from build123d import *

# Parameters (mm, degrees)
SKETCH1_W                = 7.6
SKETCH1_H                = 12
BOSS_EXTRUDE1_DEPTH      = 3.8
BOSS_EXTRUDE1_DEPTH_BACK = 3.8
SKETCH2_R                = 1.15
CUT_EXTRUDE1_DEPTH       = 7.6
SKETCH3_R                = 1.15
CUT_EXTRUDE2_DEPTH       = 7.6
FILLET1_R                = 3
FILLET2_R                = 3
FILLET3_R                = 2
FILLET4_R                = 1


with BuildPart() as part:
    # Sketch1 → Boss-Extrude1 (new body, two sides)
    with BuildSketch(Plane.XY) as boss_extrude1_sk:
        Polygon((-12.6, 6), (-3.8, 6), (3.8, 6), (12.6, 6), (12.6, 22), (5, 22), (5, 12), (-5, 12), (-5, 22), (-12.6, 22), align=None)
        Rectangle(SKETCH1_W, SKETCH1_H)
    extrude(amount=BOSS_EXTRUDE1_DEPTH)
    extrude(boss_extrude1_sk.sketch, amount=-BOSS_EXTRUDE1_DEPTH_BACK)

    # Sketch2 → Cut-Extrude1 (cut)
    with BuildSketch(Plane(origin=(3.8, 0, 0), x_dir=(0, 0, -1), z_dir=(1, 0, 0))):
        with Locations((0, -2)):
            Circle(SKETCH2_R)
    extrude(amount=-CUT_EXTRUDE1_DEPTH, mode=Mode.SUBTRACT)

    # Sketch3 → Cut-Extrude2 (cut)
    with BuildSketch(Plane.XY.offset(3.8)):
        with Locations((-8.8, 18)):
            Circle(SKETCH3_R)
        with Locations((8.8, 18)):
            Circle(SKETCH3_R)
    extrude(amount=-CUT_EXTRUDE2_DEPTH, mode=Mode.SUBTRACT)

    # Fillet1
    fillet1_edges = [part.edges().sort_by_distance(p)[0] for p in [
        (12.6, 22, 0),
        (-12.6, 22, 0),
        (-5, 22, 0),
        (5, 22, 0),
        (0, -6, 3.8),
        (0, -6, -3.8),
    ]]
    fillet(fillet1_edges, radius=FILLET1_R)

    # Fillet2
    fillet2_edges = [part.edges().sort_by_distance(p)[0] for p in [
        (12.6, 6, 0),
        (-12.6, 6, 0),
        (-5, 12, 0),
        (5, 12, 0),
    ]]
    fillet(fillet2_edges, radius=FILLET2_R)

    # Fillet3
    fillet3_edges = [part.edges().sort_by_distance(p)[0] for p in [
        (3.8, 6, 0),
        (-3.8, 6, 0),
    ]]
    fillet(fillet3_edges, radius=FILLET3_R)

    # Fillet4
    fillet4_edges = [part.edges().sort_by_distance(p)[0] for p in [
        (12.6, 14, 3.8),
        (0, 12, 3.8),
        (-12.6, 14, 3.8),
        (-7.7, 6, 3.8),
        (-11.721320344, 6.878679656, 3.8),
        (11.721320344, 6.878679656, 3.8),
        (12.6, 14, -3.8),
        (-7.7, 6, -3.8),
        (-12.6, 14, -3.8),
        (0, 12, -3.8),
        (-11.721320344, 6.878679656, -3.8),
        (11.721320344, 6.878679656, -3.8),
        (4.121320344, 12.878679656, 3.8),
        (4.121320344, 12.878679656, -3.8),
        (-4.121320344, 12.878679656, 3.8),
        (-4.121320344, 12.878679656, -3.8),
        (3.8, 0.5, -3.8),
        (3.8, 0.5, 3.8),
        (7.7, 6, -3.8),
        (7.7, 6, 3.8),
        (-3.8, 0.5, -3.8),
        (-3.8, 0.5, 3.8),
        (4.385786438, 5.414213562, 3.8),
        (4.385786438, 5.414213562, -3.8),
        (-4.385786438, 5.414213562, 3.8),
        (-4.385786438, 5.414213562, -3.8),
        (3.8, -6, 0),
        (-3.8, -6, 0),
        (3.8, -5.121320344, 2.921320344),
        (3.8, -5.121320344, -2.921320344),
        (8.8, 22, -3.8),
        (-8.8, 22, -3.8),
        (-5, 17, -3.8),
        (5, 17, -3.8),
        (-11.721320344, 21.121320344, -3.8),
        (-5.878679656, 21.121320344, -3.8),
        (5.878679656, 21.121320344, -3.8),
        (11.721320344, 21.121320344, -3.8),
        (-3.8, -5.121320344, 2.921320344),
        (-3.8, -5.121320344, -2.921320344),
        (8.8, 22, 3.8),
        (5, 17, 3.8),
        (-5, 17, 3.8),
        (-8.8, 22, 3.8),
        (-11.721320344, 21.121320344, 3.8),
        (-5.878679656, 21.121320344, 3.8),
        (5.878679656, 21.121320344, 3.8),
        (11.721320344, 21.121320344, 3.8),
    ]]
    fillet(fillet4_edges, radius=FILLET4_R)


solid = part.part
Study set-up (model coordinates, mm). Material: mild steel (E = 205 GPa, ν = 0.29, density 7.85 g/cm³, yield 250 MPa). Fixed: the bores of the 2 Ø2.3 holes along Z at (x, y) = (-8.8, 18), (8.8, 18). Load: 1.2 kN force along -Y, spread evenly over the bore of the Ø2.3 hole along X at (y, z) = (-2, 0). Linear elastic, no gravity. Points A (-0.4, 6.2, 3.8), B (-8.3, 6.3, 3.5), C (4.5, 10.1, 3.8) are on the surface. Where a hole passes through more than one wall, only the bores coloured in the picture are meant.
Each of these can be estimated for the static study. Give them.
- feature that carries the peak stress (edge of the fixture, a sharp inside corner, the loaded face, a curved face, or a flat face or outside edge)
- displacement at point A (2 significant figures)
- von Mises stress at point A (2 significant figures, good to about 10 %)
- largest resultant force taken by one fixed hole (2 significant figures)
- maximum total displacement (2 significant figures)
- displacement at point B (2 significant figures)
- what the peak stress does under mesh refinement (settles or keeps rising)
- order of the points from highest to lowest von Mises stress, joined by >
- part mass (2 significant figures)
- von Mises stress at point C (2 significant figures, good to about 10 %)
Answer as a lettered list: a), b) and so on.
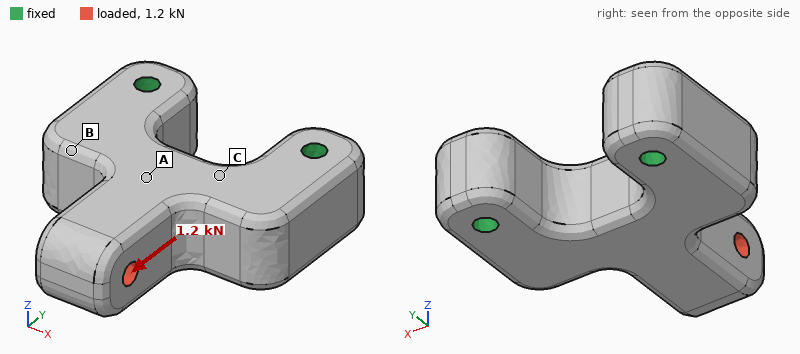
a) a sharp inside corner
b) 1.4 µm
c) 10 MPa
d) 660 N
e) 2.5 µm
f) 0.43 µm
g) keeps rising
h) C > A > B
i) 22 g
j) 23 MPa
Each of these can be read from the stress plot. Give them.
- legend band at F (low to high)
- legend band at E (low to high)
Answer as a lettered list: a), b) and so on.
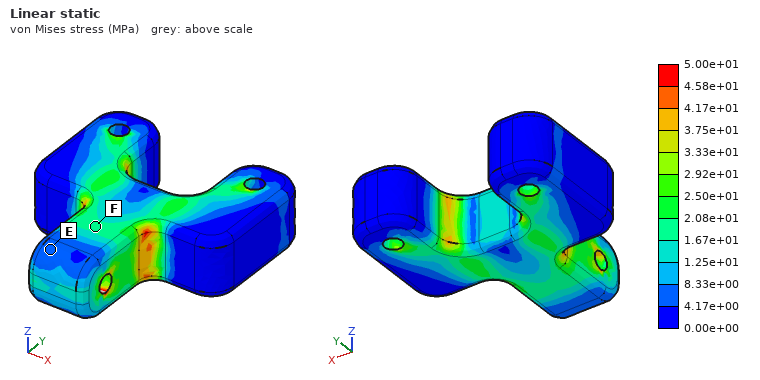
a) 1.67e+01 to 2.08e+01 MPa
b) 4.17e+00 to 8.33e+00 MPa
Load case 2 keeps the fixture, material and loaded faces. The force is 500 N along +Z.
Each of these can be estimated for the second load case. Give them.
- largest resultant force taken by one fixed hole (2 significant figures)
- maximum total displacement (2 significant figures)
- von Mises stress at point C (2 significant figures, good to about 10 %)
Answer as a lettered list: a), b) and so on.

a) 250 N
b) 25 µm
c) 64 MPa
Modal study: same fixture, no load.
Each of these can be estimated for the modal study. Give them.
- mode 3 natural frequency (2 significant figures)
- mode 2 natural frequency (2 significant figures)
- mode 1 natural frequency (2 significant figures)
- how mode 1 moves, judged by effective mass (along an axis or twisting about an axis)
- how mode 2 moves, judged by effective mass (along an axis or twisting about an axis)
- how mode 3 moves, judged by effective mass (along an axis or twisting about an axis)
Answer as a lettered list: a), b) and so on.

a) 38 kHz
b) 26 kHz
c) 12 kHz
d) along Z
e) along X
f) along X
